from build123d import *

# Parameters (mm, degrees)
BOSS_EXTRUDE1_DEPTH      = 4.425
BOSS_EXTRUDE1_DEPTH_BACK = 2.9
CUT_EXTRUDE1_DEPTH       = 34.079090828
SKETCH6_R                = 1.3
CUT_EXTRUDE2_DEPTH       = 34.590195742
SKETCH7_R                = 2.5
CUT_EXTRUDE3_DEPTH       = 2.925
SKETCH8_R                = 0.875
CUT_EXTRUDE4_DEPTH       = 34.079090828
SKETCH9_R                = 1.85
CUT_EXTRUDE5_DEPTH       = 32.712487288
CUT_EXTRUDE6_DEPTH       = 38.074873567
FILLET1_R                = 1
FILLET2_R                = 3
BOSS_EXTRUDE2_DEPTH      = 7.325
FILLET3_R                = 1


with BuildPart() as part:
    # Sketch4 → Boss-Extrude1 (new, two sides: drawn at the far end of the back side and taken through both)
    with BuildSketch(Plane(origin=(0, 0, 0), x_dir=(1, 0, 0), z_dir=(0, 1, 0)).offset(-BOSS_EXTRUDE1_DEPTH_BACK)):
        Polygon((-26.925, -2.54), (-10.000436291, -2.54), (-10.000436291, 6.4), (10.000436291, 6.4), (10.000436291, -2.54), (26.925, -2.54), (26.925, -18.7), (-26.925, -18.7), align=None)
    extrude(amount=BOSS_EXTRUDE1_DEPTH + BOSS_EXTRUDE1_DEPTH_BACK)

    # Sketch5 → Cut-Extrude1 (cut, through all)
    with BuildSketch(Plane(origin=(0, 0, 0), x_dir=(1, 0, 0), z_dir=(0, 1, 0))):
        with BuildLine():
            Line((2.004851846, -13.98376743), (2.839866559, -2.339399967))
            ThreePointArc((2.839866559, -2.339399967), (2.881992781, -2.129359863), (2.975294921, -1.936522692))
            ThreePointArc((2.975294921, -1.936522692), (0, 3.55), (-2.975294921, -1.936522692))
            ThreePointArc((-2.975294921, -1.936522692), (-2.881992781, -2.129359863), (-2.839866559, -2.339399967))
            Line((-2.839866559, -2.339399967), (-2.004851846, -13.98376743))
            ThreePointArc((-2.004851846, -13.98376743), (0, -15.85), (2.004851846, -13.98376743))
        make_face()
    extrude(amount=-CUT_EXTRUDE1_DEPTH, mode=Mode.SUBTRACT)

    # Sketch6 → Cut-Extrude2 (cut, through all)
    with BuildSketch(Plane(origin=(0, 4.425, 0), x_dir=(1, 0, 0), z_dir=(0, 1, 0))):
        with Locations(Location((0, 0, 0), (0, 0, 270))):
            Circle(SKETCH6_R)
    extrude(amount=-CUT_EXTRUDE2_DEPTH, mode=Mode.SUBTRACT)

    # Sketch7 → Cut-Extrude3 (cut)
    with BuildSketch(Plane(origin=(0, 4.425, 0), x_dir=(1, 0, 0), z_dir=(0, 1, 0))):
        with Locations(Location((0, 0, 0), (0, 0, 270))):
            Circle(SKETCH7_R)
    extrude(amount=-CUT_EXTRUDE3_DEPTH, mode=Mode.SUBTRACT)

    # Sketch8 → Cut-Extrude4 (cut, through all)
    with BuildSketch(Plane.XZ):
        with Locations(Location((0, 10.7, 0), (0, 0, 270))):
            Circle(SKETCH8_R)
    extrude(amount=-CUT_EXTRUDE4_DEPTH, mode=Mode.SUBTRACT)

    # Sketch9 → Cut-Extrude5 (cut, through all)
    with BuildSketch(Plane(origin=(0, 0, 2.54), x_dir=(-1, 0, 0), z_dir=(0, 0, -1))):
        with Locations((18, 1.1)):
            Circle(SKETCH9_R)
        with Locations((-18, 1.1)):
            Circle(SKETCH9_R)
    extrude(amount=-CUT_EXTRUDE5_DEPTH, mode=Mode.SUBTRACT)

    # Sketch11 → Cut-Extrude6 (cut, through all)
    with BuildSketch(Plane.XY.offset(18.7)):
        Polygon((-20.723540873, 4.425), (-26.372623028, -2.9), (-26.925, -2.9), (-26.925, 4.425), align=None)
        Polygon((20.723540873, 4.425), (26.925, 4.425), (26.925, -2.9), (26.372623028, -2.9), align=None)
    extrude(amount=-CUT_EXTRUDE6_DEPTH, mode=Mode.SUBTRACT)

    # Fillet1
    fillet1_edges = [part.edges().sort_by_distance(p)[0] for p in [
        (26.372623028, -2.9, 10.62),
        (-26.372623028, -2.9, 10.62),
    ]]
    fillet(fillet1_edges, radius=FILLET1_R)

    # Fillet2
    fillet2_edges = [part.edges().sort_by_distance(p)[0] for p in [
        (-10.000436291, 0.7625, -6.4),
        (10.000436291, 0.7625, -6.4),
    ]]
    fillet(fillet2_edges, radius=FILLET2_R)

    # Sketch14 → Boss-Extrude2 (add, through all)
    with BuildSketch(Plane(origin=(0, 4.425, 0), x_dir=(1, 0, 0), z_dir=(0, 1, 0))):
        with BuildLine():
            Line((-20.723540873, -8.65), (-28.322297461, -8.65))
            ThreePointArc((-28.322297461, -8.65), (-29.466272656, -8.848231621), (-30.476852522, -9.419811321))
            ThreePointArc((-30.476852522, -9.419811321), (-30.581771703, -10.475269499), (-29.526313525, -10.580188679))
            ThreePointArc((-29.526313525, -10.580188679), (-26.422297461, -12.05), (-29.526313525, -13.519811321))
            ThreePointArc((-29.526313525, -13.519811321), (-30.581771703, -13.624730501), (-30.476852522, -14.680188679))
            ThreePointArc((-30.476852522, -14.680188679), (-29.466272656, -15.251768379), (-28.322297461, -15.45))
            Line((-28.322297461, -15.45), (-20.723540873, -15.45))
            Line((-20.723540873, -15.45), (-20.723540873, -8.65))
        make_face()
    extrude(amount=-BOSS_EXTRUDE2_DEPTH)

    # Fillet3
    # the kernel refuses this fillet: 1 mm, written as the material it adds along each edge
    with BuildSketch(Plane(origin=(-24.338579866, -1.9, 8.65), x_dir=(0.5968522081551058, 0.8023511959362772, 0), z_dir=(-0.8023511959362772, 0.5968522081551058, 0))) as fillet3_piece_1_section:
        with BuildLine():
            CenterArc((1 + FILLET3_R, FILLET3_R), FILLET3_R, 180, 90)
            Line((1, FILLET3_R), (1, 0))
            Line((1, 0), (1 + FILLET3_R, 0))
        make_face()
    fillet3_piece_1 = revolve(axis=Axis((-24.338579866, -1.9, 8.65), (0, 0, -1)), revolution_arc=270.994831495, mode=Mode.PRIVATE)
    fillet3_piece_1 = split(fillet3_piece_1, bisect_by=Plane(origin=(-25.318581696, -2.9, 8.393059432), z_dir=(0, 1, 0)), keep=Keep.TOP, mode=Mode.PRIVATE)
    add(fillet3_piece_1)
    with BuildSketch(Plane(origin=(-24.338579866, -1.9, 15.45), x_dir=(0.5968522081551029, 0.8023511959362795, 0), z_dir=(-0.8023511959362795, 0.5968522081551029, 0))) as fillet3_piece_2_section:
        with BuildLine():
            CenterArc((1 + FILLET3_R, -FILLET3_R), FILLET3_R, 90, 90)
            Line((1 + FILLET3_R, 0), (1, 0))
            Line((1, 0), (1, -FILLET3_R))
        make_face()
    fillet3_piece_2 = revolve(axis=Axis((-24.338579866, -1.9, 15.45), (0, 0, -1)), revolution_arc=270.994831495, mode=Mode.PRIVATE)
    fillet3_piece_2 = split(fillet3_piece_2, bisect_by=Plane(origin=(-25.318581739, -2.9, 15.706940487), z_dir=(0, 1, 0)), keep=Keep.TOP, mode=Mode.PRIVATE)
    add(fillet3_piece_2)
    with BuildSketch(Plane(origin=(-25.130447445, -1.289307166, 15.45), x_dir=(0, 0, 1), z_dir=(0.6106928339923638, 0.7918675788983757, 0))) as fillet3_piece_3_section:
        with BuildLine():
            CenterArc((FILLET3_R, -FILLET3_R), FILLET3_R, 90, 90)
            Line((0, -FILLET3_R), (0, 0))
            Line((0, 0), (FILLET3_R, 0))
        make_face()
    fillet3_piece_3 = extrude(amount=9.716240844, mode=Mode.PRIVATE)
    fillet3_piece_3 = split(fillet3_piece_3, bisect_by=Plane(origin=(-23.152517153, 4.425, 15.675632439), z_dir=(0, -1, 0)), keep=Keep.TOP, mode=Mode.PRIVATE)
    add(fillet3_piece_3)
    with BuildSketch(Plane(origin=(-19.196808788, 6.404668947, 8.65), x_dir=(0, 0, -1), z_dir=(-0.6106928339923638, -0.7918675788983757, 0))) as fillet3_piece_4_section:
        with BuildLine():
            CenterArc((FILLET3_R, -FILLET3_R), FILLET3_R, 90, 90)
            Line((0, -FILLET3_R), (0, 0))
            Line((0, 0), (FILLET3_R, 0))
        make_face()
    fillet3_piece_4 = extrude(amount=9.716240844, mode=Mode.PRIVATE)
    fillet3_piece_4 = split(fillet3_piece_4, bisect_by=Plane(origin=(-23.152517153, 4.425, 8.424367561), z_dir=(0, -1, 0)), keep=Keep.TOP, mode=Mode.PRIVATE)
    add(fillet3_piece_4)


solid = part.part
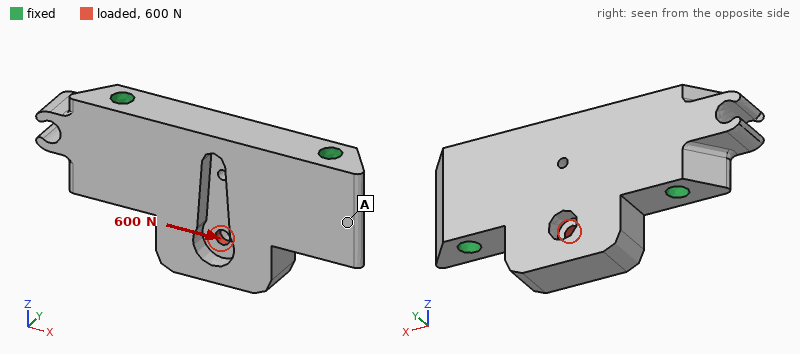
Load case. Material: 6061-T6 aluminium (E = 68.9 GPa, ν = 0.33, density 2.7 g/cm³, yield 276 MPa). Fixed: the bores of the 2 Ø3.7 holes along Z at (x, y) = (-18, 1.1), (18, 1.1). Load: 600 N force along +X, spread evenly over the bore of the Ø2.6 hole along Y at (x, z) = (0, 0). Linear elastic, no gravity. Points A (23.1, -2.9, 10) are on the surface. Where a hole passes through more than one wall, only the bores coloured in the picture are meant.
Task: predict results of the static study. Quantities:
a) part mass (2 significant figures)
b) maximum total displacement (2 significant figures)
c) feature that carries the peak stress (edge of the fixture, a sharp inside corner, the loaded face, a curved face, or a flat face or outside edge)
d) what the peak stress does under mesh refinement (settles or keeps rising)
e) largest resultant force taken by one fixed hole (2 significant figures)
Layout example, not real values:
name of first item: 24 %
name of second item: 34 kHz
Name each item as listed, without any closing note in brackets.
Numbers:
part mass: 17 g
maximum total displacement: 3.9 µm
feature that carries the peak stress: a sharp inside corner
what the peak stress does under mesh refinement: keeps rising
largest resultant force taken by one fixed hole: 340 N
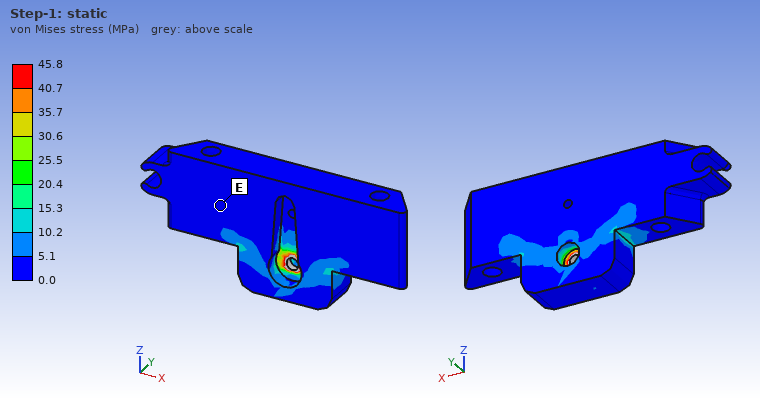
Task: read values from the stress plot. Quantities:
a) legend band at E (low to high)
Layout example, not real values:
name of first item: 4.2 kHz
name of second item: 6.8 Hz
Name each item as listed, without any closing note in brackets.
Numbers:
legend band at E: 0.0 to 5.1 MPa
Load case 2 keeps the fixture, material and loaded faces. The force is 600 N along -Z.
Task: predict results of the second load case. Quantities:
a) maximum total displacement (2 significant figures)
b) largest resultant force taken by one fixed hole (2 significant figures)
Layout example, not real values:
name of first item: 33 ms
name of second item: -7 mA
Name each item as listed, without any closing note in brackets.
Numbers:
maximum total displacement: 4.0 µm
largest resultant force taken by one fixed hole: 320 N
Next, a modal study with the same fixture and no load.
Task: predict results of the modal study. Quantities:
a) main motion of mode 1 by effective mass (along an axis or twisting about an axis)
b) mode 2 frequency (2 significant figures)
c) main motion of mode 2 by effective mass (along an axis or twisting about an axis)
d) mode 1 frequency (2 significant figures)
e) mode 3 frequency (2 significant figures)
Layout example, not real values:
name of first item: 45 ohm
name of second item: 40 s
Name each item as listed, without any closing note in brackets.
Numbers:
main motion of mode 1 by effective mass: along Y
mode 2 frequency: 25 kHz
main motion of mode 2 by effective mass: along Y
mode 1 frequency: 15 kHz
mode 3 frequency: 33 kHz
